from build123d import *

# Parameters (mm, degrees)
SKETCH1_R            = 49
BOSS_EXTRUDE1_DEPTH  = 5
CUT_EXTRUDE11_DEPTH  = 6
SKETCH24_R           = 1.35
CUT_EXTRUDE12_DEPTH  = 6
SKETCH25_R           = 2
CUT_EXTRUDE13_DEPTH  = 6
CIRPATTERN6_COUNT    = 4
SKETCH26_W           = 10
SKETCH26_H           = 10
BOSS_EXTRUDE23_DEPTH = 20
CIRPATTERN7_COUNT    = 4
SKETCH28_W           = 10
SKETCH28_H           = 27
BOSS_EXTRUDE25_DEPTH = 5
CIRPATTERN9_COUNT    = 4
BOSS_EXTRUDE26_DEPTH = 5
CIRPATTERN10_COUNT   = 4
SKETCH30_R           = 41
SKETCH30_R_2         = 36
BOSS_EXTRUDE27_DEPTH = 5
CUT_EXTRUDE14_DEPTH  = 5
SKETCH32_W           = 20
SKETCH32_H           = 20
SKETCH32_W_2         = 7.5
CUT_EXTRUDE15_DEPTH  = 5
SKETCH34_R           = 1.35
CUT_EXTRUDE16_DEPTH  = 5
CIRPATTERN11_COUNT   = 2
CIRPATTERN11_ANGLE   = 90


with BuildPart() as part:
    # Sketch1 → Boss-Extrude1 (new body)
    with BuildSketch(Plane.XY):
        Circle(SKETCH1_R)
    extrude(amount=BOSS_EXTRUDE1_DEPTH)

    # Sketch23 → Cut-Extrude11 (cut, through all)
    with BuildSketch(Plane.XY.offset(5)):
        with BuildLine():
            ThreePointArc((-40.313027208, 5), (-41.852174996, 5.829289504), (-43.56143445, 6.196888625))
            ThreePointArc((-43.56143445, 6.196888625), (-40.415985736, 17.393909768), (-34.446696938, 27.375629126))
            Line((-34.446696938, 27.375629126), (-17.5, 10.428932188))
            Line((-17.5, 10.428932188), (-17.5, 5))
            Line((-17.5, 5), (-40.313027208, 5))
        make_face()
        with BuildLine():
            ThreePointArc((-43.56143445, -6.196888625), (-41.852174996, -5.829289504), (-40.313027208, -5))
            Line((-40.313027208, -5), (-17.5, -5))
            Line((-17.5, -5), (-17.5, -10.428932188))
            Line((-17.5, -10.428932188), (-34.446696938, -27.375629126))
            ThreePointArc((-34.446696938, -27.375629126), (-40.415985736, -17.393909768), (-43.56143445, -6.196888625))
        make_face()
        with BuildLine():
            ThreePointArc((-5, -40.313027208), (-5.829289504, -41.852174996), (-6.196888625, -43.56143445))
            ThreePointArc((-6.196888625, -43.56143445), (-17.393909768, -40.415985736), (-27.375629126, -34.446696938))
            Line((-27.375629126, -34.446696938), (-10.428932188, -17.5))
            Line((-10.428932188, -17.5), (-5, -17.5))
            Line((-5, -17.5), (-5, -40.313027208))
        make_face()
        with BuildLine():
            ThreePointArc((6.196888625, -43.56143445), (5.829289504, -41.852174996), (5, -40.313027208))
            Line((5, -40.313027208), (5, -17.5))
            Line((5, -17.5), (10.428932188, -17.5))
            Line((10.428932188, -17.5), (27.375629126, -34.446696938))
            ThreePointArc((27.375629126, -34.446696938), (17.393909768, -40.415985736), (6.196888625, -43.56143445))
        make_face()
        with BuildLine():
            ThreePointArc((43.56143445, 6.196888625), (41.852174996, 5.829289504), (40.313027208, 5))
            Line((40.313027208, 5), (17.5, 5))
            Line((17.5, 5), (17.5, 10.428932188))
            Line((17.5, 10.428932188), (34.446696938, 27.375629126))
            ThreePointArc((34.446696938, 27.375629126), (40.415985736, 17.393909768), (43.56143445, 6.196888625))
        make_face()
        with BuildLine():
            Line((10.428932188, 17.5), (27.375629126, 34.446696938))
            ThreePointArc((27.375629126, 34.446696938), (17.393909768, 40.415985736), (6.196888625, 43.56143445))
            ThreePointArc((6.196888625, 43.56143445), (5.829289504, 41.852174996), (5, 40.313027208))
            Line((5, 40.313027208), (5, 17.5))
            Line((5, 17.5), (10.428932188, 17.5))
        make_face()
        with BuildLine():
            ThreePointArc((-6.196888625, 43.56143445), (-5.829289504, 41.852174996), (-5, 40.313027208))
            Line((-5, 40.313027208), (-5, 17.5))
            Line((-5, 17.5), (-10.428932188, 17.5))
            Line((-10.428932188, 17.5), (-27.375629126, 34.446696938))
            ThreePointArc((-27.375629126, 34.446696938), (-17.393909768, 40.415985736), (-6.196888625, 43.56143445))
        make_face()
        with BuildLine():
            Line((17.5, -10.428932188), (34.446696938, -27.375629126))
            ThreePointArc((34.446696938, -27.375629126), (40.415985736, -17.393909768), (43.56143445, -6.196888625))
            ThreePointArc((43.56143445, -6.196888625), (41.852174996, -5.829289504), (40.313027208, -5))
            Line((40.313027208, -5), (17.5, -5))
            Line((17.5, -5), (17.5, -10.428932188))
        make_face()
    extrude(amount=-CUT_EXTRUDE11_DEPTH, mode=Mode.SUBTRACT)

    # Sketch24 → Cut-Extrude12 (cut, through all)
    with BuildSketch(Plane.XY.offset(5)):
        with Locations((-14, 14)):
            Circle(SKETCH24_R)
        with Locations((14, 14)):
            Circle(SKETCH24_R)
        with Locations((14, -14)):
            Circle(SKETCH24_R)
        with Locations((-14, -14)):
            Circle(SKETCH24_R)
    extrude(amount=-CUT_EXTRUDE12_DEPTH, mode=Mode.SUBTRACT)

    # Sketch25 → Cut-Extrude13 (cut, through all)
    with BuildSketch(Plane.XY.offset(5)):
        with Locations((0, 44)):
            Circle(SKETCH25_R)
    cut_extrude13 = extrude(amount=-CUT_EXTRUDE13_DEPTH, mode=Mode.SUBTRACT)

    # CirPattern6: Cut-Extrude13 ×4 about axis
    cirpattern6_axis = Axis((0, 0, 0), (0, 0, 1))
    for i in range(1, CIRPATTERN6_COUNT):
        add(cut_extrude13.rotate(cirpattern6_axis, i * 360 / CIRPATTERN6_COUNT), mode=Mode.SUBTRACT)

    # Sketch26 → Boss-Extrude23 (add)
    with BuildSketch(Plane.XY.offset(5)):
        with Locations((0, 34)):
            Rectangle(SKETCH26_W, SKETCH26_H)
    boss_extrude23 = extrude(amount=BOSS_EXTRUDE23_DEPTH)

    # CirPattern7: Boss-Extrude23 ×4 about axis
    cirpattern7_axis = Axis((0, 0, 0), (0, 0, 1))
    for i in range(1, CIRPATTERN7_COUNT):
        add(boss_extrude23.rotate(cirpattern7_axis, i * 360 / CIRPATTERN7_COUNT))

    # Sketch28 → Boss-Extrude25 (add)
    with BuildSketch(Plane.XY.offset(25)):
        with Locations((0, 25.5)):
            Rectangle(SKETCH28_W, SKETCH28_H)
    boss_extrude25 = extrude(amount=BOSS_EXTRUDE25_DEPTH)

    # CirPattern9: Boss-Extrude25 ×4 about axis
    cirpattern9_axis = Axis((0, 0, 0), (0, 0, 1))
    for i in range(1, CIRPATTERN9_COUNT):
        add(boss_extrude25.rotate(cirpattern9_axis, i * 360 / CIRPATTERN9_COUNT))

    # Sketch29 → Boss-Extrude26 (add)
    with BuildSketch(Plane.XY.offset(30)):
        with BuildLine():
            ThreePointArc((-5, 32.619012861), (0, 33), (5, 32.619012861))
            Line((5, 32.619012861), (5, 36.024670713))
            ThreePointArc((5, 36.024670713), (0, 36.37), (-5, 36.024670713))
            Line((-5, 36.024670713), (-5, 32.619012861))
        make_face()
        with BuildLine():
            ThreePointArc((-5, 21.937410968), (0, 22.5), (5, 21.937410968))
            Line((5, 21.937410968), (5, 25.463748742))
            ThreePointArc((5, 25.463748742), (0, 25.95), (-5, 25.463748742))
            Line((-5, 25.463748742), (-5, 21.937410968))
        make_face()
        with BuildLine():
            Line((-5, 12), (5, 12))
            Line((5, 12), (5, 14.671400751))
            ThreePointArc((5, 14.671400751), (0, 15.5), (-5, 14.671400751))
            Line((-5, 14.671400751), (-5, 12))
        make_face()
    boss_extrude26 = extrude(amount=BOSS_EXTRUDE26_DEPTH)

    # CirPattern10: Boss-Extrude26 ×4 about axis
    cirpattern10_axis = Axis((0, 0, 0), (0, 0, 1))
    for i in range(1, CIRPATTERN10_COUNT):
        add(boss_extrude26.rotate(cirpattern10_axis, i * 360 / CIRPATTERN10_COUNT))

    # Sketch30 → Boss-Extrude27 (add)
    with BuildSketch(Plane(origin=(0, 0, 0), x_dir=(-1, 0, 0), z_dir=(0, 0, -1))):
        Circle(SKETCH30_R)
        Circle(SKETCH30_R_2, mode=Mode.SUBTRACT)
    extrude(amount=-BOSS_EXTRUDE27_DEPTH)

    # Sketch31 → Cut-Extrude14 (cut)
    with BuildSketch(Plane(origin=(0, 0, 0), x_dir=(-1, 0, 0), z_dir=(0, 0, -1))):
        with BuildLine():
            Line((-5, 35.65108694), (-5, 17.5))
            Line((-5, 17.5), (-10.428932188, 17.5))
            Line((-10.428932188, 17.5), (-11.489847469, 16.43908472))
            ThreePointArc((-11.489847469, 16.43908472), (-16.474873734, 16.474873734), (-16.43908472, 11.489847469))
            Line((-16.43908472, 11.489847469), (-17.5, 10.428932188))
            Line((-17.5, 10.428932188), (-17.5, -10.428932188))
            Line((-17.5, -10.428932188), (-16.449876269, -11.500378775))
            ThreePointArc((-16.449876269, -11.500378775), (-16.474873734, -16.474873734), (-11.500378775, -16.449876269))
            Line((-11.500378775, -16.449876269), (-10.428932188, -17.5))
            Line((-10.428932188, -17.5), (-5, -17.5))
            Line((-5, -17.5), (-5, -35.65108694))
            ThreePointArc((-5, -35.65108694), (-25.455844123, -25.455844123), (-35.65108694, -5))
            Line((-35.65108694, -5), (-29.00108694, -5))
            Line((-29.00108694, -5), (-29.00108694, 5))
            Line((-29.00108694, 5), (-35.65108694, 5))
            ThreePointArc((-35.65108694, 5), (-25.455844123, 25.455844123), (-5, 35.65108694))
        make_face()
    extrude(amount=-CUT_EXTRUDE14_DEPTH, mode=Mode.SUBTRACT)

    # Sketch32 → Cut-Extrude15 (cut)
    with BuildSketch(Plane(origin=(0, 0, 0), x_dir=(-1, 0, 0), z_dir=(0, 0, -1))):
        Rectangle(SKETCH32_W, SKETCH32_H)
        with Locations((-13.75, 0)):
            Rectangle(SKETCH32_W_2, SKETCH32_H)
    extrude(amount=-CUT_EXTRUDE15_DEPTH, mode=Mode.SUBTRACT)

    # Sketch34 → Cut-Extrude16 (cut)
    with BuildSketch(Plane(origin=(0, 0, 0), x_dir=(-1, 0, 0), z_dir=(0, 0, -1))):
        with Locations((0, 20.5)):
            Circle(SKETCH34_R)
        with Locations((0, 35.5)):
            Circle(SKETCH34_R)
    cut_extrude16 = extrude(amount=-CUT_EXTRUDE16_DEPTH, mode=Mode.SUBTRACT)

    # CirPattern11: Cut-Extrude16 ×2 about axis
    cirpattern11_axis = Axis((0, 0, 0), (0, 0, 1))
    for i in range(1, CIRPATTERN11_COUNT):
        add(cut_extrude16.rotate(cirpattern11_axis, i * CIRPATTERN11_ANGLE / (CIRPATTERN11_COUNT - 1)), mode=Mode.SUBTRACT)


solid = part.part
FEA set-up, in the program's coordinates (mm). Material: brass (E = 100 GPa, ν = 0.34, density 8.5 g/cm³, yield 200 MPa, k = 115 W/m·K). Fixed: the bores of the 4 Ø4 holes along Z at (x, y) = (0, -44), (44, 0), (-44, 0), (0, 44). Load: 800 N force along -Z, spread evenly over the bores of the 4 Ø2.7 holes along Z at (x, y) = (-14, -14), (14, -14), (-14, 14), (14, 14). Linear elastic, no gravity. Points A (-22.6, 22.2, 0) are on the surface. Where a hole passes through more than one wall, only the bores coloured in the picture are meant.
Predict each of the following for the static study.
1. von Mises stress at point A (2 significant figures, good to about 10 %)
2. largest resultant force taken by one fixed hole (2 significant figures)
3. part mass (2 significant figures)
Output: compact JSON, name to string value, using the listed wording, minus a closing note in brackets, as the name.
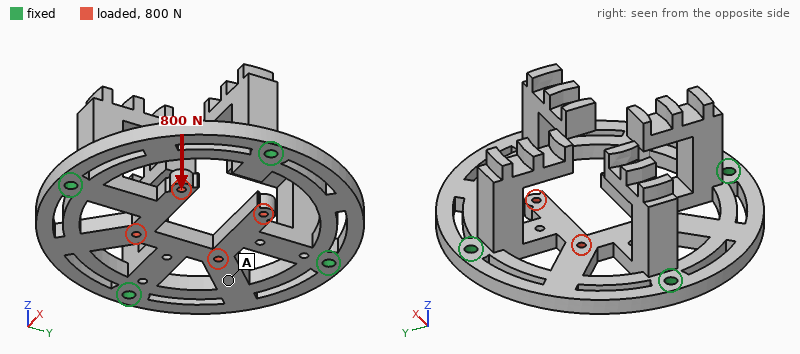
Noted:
{"von Mises stress at point A": "17 MPa", "largest resultant force taken by one fixed hole": "300 N", "part mass": "320 g"}
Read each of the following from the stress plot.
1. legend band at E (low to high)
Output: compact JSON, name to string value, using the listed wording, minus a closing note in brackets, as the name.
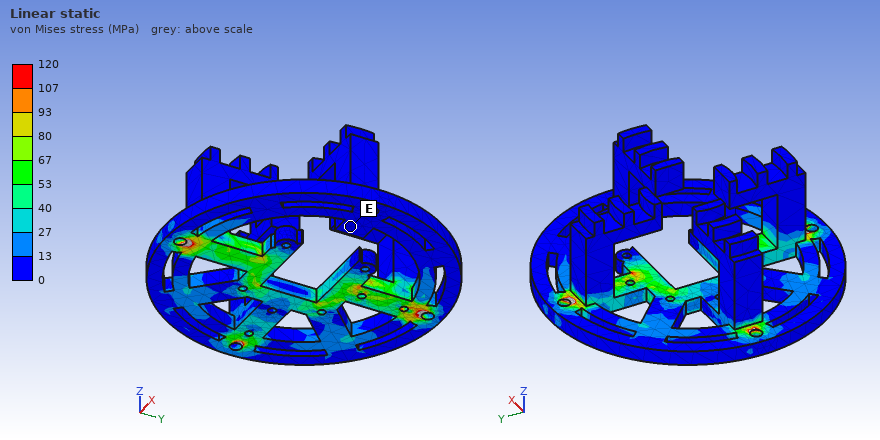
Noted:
{"legend band at E": "0 to 13 MPa"}
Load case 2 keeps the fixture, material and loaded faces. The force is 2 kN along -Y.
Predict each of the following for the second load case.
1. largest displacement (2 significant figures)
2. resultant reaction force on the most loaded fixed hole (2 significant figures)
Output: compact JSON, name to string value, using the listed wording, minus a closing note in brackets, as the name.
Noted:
{"largest displacement": "48 µm", "resultant reaction force on the most loaded fixed hole": "870 N"}
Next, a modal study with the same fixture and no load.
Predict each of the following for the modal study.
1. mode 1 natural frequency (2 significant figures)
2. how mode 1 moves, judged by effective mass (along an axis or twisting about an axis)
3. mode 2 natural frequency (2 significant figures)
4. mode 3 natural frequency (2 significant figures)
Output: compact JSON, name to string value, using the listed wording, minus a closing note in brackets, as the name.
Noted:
{"mode 1 natural frequency": "1400 Hz", "how mode 1 moves, judged by effective mass": "along Z", "mode 2 natural frequency": "1500 Hz", "mode 3 natural frequency": "1700 Hz"}
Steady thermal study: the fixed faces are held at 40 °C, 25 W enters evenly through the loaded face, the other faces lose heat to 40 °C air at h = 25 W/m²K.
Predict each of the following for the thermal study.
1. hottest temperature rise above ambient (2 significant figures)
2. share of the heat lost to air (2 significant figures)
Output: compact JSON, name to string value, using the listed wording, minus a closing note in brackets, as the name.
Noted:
{"hottest temperature rise above ambient": "44 K", "share of the heat lost to air": "17 %"}
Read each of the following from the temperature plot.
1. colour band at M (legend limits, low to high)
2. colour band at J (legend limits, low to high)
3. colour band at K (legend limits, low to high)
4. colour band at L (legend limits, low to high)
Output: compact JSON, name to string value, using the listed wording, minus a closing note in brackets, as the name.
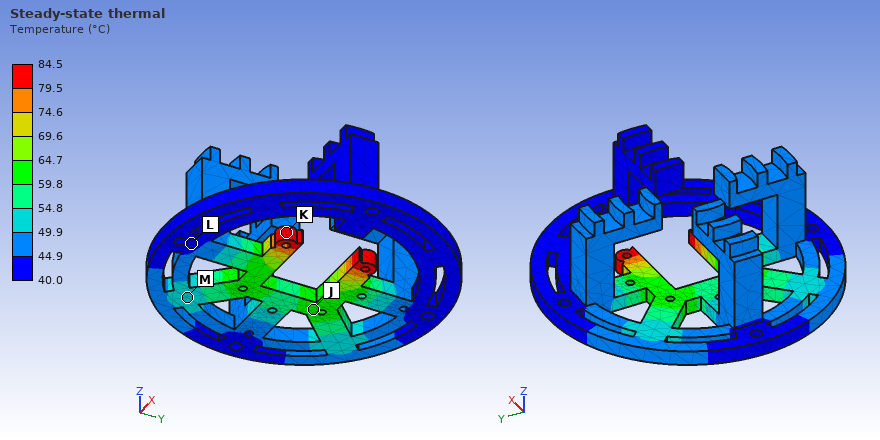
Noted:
{"colour band at M": "49.9 to 54.8 °C", "colour band at J": "59.8 to 64.7 °C", "colour band at K": "79.5 to 84.5 °C", "colour band at L": "40.0 to 44.9 °C"}
